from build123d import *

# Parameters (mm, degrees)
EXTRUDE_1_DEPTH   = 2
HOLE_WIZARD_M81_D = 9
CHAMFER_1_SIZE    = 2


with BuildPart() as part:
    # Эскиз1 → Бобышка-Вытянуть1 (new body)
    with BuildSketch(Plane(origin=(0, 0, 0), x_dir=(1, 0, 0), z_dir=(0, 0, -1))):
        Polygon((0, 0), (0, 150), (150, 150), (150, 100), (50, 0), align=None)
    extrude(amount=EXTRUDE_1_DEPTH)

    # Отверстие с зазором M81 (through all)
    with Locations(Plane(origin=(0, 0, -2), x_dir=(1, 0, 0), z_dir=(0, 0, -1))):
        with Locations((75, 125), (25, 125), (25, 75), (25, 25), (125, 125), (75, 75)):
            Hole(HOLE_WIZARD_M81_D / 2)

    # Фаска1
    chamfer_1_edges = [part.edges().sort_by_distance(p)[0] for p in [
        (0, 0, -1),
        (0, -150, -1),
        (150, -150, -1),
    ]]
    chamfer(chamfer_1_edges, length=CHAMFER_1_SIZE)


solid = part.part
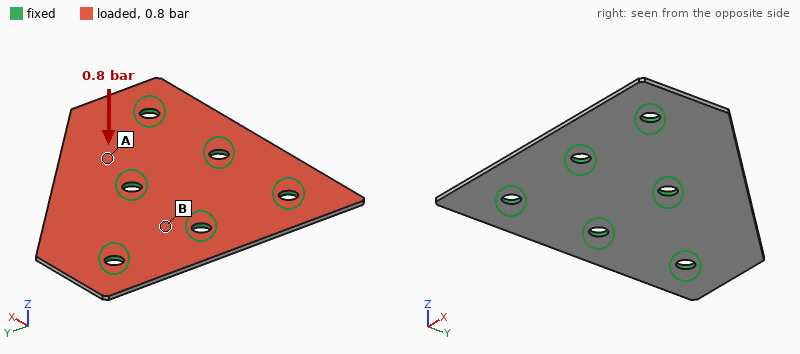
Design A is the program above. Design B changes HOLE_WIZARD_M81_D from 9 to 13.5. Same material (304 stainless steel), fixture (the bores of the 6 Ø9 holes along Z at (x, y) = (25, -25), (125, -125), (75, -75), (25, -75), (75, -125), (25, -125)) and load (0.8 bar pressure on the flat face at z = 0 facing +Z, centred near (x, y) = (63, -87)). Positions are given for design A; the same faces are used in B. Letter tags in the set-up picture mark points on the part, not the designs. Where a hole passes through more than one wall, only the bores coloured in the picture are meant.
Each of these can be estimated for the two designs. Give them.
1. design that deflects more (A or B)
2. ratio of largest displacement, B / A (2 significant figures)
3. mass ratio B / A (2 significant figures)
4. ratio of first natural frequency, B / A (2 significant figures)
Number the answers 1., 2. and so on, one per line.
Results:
1. A
2. 0.78
3. 0.97
4. 1.1
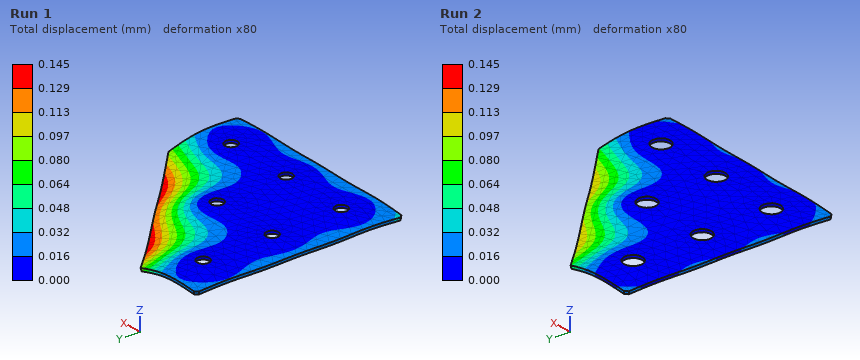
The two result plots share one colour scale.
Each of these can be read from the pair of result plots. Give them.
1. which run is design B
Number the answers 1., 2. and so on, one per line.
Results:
1. Run 2
